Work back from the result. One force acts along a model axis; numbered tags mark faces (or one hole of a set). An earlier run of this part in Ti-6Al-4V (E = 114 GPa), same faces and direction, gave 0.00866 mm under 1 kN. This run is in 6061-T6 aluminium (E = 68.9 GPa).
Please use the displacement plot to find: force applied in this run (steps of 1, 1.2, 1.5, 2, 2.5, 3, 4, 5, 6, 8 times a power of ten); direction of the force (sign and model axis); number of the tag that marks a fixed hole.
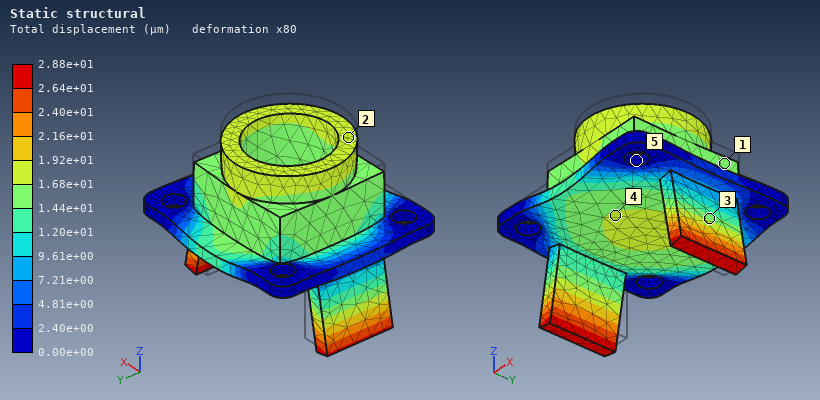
2 kN
-Z
5
